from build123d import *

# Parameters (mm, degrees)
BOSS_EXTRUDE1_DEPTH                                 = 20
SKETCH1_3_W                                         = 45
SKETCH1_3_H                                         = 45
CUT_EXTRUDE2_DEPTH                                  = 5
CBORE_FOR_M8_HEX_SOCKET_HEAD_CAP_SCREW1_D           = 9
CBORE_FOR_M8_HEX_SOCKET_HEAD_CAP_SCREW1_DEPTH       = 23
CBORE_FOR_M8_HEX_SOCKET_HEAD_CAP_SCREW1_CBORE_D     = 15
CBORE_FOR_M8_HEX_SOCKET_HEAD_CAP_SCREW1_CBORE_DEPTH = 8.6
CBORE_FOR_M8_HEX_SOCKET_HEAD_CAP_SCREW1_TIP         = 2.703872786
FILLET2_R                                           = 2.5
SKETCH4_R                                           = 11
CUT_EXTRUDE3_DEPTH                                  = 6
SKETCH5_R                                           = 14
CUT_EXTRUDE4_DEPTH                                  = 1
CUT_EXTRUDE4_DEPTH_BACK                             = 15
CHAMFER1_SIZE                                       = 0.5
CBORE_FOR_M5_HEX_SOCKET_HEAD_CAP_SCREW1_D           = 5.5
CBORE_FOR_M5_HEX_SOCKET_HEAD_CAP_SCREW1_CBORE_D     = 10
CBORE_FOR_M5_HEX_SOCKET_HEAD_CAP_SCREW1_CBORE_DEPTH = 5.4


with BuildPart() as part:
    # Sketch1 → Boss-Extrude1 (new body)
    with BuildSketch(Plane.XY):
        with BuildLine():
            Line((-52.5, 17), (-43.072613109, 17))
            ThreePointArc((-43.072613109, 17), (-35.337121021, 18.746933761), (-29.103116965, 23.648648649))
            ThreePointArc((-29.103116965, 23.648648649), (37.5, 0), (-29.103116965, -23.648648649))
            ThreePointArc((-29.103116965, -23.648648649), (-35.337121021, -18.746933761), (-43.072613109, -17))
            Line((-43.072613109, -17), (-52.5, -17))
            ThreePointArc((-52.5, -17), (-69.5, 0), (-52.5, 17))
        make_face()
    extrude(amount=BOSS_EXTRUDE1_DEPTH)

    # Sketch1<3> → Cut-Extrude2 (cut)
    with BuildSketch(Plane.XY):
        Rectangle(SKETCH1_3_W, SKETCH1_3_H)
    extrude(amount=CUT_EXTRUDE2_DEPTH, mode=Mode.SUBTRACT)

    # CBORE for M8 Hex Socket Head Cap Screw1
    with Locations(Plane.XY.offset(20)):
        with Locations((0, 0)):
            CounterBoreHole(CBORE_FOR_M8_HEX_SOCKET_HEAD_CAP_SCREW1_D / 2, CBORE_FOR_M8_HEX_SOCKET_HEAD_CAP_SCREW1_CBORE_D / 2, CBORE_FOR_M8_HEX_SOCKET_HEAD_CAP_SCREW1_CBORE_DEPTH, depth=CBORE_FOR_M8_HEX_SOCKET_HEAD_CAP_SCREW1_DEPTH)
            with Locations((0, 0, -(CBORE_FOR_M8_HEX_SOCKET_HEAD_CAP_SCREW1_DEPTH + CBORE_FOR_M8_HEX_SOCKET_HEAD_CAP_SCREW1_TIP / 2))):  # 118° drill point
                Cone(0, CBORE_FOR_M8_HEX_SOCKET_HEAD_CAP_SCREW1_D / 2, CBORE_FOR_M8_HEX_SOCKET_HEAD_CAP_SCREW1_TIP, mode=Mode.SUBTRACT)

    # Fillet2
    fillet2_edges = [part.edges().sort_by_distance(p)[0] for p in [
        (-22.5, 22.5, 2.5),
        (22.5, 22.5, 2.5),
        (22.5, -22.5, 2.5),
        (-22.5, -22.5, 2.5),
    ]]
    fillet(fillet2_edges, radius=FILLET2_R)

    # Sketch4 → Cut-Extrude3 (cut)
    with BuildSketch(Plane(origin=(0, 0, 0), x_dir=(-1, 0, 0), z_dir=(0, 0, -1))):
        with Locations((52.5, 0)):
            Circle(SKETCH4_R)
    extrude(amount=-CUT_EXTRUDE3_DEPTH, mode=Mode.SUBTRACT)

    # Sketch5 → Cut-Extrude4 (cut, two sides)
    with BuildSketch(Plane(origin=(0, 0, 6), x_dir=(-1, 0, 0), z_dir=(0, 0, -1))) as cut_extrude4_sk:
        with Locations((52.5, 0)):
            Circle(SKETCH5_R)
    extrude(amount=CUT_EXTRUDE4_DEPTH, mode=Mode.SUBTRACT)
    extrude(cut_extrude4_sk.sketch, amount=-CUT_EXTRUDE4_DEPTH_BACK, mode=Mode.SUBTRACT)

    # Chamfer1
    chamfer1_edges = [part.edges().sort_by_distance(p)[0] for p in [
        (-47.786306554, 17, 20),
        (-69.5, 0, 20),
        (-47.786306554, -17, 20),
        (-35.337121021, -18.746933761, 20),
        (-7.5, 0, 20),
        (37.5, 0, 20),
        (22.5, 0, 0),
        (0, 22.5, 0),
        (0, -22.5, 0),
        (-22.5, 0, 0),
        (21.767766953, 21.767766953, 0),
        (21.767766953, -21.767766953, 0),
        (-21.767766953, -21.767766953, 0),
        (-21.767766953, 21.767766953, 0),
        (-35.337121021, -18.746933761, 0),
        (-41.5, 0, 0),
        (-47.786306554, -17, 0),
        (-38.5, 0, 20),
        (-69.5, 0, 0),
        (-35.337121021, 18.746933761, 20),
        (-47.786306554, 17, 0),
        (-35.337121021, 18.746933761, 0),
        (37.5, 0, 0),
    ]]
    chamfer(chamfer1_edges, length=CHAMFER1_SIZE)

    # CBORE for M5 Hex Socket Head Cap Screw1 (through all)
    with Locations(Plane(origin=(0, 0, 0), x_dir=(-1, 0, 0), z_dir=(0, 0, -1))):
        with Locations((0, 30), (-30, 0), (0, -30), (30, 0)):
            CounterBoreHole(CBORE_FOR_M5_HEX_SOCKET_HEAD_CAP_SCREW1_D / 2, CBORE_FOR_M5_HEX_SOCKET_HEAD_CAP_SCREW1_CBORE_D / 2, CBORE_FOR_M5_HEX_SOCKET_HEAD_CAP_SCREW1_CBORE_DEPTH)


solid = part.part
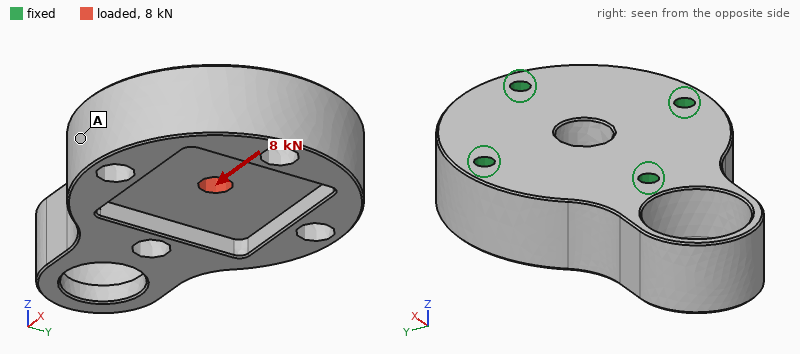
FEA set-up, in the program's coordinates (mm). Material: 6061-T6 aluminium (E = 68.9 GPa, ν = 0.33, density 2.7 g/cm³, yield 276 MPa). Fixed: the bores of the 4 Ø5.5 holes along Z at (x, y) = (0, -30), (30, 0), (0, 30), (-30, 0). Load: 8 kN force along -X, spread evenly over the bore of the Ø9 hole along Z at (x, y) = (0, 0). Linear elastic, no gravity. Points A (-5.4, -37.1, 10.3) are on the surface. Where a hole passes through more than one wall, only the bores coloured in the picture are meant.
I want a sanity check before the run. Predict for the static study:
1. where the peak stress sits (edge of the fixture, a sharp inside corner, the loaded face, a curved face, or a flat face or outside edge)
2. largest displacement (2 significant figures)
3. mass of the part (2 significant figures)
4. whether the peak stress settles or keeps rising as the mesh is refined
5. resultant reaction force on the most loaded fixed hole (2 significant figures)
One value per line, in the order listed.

a sharp inside corner
8.7 µm
220 g
keeps rising
2.7 kN
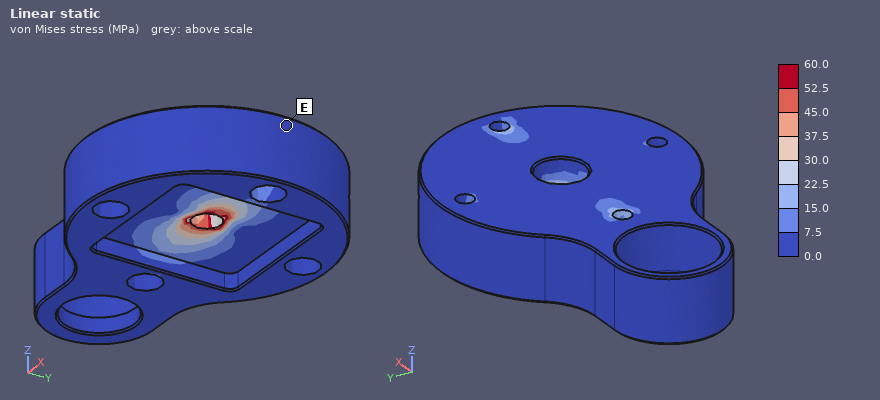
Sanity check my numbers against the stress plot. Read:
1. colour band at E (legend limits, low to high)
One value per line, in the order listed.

0.0 to 7.5 MPa
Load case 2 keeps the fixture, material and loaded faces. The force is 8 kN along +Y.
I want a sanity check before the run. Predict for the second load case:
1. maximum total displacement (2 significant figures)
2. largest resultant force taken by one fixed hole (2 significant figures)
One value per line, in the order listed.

8.7 µm
2.7 kN
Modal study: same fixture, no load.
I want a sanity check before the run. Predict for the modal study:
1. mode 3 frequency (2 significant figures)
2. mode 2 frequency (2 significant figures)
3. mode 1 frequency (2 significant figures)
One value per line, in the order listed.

13 kHz
8100 Hz
7700 Hz
